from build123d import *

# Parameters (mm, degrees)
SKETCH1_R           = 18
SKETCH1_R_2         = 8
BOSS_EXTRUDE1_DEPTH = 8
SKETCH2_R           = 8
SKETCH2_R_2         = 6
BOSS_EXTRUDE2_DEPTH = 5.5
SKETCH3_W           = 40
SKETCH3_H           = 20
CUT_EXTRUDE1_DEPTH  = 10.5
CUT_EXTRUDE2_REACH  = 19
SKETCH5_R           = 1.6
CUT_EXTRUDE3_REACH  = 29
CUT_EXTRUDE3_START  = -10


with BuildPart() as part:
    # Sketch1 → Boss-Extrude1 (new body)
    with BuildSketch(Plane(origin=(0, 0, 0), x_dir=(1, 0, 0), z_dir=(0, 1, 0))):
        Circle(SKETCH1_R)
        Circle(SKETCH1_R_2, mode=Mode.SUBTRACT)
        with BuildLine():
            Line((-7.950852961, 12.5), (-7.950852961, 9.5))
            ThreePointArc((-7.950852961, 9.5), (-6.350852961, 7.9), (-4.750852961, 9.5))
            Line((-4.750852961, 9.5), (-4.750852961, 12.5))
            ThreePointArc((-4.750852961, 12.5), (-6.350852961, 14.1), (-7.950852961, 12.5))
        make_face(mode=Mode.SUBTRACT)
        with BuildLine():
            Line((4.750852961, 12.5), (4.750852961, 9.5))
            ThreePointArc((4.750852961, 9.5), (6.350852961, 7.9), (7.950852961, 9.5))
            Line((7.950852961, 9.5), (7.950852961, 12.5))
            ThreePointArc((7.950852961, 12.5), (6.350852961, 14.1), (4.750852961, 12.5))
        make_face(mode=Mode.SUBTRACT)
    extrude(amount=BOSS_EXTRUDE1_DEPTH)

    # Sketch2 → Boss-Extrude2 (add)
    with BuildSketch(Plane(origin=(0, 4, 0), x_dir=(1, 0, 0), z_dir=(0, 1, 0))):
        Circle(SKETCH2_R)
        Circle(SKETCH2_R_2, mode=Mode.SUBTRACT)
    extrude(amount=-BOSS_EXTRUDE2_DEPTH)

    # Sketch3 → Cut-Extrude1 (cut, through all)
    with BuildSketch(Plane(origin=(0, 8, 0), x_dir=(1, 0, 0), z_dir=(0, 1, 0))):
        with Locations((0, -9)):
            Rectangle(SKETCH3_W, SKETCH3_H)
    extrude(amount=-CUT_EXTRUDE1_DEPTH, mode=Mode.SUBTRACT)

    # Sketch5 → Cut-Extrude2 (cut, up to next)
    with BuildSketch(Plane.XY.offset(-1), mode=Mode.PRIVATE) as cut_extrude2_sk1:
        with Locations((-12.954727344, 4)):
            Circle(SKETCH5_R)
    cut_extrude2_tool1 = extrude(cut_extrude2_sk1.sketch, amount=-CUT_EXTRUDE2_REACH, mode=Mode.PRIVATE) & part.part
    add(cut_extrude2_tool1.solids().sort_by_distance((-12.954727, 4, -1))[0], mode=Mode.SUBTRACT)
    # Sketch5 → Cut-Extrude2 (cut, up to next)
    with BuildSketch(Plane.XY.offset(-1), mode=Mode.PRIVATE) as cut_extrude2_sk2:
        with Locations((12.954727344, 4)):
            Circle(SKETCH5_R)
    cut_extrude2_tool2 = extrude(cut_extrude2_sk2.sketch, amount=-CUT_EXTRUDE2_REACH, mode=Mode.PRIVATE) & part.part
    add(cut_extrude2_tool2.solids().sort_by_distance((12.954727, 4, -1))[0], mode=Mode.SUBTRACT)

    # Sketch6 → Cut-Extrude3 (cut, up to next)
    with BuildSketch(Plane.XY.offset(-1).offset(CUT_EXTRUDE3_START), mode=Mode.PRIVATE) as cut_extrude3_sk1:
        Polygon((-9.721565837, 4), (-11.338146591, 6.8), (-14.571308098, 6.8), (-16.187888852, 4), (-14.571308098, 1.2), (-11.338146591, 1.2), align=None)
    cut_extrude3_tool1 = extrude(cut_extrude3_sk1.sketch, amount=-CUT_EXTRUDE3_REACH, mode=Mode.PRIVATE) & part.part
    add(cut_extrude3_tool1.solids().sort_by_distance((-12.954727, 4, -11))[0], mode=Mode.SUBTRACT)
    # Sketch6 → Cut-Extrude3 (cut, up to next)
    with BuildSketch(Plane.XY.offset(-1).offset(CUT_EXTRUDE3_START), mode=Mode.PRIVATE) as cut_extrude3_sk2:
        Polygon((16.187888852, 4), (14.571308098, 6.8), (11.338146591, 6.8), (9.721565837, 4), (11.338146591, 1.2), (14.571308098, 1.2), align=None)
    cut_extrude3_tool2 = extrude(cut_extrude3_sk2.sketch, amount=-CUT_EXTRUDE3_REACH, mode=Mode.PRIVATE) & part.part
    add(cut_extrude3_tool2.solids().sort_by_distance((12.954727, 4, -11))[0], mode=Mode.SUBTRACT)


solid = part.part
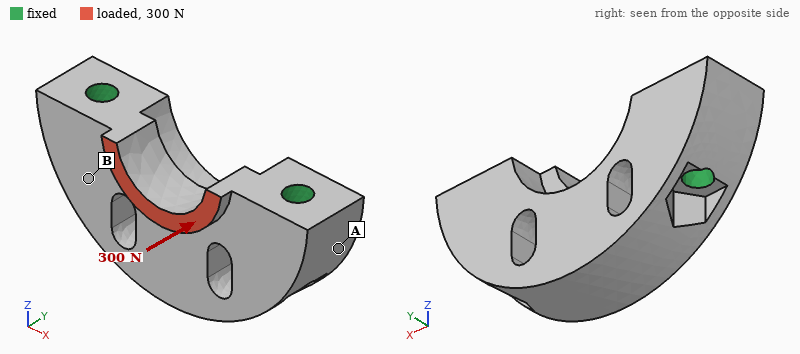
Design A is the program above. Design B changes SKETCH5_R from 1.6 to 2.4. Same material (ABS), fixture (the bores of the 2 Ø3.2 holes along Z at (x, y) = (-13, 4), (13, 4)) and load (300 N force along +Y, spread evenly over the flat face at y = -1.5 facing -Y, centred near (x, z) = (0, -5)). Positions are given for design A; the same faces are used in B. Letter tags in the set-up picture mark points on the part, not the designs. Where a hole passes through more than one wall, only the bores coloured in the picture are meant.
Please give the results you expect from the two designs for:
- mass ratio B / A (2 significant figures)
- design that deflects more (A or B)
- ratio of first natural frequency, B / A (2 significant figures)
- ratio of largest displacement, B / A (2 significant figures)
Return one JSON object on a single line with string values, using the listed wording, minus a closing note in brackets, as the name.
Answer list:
{"mass ratio B / A": "0.93", "design that deflects more": "A", "ratio of first natural frequency, B / A": "1.1", "ratio of largest displacement, B / A": "0.79"}
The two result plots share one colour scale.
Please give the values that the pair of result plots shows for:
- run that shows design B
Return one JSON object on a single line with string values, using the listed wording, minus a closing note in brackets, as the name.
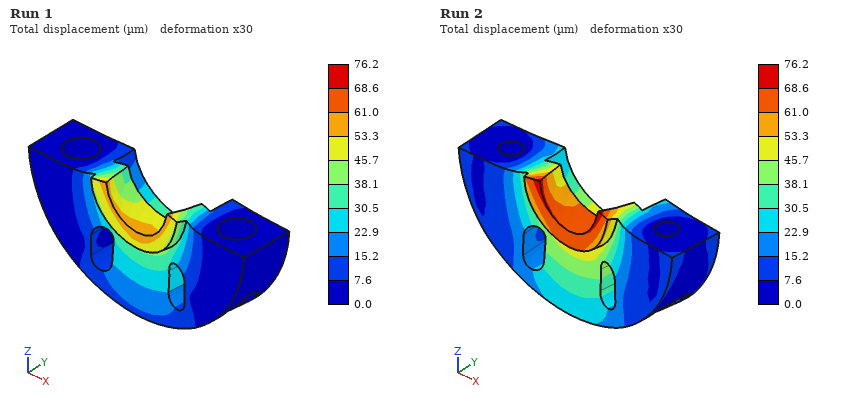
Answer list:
{"run that shows design B": "Run 1"}
